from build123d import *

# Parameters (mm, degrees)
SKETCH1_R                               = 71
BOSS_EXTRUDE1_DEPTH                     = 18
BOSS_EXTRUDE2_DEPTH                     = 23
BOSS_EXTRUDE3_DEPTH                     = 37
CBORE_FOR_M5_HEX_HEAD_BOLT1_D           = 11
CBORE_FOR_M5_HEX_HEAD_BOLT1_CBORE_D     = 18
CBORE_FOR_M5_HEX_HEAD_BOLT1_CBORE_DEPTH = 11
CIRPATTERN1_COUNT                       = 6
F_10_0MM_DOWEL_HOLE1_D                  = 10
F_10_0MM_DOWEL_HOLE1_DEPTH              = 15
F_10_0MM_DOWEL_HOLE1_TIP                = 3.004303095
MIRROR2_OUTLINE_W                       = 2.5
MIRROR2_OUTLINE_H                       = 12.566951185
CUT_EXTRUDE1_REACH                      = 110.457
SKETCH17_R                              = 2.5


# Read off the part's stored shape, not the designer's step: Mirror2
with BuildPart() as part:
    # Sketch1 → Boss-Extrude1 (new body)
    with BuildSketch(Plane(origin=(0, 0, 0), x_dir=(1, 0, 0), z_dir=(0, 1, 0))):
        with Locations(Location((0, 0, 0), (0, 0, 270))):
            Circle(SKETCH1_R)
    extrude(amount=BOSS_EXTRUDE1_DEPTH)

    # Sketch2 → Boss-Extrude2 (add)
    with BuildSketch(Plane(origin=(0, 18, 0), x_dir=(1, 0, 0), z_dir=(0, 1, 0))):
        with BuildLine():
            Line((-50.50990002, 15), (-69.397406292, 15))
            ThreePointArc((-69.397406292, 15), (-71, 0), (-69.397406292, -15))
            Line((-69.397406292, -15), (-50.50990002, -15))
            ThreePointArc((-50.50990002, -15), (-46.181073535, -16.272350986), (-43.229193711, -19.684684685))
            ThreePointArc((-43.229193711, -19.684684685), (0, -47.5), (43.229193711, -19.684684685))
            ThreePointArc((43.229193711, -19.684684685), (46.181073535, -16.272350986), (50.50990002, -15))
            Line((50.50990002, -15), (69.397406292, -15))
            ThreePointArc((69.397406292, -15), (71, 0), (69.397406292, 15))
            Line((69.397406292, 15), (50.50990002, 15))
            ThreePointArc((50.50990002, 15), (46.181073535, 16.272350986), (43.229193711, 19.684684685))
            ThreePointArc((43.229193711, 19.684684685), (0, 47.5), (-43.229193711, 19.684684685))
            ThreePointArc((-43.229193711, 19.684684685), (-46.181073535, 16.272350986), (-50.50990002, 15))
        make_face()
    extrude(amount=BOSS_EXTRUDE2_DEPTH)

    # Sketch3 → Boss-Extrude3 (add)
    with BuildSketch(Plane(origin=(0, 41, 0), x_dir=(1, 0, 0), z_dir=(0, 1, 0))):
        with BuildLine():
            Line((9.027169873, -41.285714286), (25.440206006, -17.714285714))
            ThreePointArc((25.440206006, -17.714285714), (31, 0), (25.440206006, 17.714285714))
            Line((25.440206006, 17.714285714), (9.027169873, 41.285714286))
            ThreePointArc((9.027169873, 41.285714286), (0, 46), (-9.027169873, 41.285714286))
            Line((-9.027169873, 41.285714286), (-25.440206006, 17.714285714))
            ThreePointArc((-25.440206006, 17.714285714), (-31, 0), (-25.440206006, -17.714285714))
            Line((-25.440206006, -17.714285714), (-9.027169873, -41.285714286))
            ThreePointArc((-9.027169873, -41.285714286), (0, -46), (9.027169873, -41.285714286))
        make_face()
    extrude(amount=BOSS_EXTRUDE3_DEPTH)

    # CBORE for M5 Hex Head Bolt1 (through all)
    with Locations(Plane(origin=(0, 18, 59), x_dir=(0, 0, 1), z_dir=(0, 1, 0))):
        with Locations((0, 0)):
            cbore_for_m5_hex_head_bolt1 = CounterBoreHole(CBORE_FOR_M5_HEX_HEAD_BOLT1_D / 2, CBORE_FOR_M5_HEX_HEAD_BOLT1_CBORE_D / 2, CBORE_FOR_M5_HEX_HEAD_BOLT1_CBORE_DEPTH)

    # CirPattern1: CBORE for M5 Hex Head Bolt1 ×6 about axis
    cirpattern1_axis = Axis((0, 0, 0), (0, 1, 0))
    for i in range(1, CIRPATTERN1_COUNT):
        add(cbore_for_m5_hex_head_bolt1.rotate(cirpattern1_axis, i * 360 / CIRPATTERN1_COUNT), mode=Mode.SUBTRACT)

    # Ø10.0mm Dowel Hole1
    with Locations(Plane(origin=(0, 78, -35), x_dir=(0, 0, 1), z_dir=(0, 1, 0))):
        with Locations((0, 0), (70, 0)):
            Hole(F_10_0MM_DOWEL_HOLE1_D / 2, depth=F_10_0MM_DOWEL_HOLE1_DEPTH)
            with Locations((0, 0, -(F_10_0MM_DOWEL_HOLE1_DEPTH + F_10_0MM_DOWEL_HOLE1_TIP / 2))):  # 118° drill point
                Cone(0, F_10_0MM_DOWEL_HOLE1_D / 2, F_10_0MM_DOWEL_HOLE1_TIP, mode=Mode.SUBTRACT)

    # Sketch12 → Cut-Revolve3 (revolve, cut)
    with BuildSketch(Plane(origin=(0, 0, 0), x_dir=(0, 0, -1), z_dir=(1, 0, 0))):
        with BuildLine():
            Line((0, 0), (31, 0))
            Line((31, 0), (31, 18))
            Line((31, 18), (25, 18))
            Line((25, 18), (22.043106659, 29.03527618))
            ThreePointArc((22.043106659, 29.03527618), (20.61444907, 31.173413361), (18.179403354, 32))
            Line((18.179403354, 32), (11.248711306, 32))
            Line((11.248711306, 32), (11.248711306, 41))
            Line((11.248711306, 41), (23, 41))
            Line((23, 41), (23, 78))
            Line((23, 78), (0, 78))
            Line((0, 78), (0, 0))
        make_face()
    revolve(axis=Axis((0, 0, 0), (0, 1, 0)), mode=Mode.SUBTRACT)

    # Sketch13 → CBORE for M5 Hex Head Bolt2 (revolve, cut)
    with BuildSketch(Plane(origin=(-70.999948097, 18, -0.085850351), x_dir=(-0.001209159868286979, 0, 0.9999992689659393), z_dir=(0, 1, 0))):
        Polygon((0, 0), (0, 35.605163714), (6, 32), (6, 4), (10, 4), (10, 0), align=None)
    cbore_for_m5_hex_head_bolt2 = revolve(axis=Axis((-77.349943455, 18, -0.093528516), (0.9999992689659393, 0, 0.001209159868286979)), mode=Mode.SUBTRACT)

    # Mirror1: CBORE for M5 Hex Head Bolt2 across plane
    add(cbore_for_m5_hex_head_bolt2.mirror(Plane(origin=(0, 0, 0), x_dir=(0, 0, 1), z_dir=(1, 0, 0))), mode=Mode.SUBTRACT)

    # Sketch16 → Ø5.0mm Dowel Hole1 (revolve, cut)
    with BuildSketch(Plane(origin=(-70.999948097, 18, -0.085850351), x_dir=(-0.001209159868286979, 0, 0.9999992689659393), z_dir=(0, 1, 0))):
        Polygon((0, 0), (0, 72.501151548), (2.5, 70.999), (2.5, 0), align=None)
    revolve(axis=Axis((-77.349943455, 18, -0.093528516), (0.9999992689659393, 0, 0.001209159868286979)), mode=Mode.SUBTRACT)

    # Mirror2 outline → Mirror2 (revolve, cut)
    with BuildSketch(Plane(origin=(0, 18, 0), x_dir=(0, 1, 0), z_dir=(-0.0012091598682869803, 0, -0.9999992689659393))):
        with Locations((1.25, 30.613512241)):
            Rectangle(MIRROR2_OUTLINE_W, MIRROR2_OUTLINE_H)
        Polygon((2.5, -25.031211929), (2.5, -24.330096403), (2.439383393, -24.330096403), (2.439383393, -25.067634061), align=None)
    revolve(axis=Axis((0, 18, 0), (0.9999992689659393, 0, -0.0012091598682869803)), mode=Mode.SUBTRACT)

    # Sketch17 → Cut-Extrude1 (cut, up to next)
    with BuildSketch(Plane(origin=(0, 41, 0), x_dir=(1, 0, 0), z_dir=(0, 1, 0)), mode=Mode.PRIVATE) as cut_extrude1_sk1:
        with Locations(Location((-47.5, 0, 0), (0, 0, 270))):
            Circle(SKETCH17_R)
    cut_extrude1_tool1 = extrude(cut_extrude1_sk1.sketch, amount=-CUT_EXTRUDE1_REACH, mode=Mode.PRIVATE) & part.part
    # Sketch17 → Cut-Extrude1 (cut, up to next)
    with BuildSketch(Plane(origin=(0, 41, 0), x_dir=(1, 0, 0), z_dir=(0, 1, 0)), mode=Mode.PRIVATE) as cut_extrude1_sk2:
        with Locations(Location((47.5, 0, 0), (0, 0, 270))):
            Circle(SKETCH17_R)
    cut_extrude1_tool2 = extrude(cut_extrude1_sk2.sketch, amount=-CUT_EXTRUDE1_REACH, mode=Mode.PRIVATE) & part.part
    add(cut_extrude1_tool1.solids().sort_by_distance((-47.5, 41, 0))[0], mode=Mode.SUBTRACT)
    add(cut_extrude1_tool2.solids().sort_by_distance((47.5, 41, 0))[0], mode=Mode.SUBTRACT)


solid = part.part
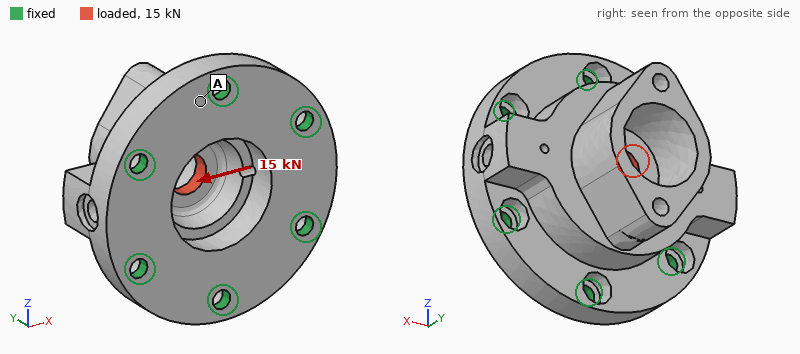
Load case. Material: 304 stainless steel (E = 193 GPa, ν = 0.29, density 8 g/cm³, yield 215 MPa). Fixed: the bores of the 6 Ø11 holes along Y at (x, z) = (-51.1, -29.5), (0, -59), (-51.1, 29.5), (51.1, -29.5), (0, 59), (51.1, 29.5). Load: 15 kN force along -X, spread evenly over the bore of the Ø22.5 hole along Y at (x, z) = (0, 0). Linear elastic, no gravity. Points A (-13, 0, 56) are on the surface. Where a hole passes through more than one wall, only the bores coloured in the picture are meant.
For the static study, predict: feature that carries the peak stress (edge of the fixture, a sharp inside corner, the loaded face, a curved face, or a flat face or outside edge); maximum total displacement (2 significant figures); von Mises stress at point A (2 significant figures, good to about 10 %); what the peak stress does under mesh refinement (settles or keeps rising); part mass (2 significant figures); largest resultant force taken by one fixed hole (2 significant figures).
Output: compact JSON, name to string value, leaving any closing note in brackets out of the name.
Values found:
{"feature that carries the peak stress": "edge of the fixture", "maximum total displacement": "5.6 µm", "von Mises stress at point A": "5.9 MPa", "what the peak stress does under mesh refinement": "keeps rising", "part mass": "3.6 kg", "largest resultant force taken by one fixed hole": "3.7 kN"}
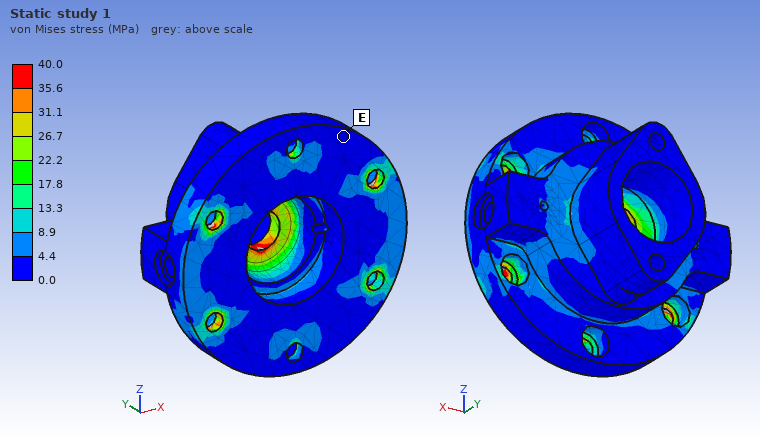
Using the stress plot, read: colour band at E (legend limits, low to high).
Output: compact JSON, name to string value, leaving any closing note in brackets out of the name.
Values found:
{"colour band at E": "0.0 to 4.4 MPa"}
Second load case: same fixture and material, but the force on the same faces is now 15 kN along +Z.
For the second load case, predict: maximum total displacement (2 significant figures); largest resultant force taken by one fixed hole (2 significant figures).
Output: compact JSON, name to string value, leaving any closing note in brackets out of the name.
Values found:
{"maximum total displacement": "5.6 µm", "largest resultant force taken by one fixed hole": "4.2 kN"}
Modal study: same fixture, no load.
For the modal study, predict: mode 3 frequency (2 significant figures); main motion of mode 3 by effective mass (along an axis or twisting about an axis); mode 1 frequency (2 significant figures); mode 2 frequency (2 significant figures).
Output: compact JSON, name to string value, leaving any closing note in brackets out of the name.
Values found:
{"mode 3 frequency": "7800 Hz", "main motion of mode 3 by effective mass": "along Y", "mode 1 frequency": "6600 Hz", "mode 2 frequency": "6600 Hz"}
